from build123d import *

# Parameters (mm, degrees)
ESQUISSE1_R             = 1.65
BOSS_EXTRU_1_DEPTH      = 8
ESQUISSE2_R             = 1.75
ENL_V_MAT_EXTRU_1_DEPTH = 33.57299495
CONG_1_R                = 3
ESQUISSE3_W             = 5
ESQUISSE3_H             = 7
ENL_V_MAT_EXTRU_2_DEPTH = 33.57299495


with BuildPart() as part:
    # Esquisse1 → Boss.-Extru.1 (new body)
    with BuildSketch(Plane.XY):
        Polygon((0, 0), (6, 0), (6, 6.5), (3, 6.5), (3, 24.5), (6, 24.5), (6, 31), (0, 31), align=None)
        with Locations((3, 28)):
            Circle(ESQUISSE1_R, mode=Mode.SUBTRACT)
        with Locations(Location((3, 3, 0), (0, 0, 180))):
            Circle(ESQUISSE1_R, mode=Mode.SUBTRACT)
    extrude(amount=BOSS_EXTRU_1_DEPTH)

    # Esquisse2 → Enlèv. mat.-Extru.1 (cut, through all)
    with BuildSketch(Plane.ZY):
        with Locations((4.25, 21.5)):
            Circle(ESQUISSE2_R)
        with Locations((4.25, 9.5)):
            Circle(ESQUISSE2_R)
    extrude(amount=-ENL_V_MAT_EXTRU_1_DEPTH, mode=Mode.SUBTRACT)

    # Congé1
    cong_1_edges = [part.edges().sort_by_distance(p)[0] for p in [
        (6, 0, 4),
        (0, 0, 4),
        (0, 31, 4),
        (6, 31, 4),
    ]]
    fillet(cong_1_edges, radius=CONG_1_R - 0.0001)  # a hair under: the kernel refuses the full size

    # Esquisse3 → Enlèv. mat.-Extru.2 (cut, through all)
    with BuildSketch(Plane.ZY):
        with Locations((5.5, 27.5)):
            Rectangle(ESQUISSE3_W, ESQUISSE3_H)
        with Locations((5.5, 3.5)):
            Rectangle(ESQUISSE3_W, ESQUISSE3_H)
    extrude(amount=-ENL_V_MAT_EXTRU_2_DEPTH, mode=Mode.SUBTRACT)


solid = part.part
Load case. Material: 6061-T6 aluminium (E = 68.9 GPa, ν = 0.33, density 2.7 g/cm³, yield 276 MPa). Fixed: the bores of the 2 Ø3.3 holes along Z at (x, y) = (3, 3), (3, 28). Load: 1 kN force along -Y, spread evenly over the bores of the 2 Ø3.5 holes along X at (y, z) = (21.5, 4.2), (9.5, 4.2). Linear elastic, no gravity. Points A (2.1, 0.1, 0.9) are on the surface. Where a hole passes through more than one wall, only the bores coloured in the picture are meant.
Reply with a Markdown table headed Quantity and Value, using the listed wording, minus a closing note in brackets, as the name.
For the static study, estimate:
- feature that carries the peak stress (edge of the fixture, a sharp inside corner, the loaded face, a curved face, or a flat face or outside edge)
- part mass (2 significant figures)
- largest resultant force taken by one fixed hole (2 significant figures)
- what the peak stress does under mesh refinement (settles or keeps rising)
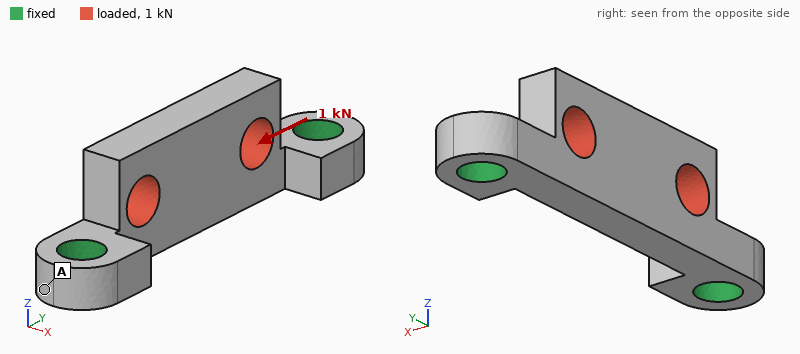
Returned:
| Quantity | Value |
|---|---|
| feature that carries the peak stress | a sharp inside corner |
| part mass | 1.4 g |
| largest resultant force taken by one fixed hole | 520 N |
| what the peak stress does under mesh refinement | keeps rising |
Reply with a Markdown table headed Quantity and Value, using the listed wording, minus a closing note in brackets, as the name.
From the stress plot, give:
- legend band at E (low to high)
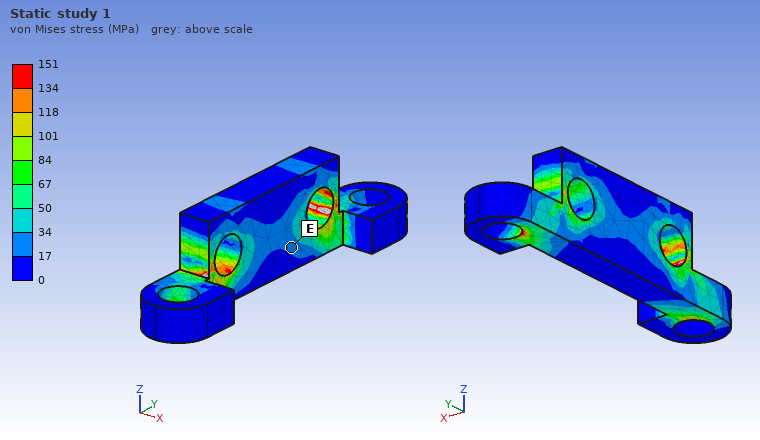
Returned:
| Quantity | Value |
|---|---|
| legend band at E | 17 to 34 MPa |
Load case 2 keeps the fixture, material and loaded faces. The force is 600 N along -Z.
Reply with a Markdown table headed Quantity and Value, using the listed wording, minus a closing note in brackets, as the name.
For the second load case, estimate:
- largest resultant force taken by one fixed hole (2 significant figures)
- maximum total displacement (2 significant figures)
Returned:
| Quantity | Value |
|---|---|
| largest resultant force taken by one fixed hole | 310 N |
| maximum total displacement | 20 µm |
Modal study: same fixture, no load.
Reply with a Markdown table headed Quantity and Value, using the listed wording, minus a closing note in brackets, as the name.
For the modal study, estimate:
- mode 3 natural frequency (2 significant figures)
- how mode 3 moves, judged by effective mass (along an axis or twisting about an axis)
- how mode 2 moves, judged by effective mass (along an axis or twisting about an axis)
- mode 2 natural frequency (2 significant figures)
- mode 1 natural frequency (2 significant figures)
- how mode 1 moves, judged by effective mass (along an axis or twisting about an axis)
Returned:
| Quantity | Value |
|---|---|
| mode 3 natural frequency | 34 kHz |
| how mode 3 moves, judged by effective mass | along X |
| how mode 2 moves, judged by effective mass | along Z |
| mode 2 natural frequency | 28 kHz |
| mode 1 natural frequency | 15 kHz |
| how mode 1 moves, judged by effective mass | along X |
